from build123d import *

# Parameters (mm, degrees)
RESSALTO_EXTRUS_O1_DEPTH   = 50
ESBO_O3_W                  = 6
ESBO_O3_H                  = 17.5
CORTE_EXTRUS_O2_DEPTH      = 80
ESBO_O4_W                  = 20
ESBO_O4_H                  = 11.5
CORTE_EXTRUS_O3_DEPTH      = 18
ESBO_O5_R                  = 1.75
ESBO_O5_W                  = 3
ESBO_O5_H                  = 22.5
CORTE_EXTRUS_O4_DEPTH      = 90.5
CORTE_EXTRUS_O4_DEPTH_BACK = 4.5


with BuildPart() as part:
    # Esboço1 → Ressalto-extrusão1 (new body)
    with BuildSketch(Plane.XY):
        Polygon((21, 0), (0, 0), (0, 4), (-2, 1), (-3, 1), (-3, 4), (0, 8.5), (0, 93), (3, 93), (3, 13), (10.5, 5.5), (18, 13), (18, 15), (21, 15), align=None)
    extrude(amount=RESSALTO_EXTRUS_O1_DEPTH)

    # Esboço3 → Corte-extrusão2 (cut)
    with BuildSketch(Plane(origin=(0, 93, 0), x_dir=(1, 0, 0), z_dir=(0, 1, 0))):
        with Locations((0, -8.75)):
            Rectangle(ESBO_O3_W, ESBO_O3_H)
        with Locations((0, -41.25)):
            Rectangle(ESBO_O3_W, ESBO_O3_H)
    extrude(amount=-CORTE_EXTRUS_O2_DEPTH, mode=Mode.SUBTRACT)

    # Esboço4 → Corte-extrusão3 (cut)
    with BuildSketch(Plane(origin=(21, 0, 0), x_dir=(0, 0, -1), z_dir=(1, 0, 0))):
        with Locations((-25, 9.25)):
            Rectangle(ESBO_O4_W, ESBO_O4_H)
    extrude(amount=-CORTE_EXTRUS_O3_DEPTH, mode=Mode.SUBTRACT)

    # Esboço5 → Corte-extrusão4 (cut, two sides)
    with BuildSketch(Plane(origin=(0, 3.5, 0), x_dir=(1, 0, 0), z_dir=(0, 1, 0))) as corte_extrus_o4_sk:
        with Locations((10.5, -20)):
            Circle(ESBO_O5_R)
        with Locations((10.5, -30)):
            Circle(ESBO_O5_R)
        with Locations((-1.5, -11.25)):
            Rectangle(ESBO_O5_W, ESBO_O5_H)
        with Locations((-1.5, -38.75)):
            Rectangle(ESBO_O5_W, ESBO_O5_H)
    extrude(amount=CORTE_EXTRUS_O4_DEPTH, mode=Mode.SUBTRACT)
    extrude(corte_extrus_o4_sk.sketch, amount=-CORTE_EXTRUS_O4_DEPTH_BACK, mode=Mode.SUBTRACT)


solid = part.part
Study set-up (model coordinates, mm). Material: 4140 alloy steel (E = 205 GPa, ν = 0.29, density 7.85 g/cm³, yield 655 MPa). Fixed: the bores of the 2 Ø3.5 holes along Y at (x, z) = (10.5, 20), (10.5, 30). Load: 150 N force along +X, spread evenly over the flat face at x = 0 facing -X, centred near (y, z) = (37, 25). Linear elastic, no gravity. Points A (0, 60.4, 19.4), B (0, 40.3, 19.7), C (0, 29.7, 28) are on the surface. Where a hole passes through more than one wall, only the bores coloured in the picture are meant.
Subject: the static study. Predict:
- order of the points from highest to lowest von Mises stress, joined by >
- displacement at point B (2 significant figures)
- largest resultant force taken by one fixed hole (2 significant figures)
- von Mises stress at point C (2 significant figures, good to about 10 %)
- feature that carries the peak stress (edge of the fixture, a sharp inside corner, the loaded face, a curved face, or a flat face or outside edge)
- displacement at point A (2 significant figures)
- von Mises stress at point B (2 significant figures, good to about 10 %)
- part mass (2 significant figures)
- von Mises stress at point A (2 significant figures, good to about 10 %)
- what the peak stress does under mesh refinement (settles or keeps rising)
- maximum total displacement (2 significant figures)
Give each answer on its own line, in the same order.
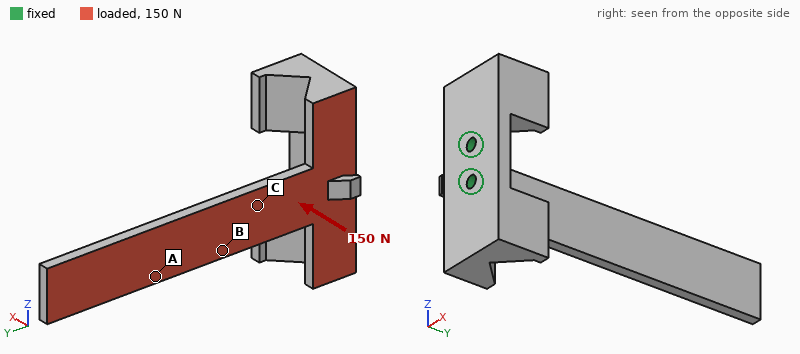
C > B > A
0.29 mm
77 N
110 MPa
a sharp inside corner
0.62 mm
76 MPa
97 g
29 MPa
keeps rising
1.2 mm
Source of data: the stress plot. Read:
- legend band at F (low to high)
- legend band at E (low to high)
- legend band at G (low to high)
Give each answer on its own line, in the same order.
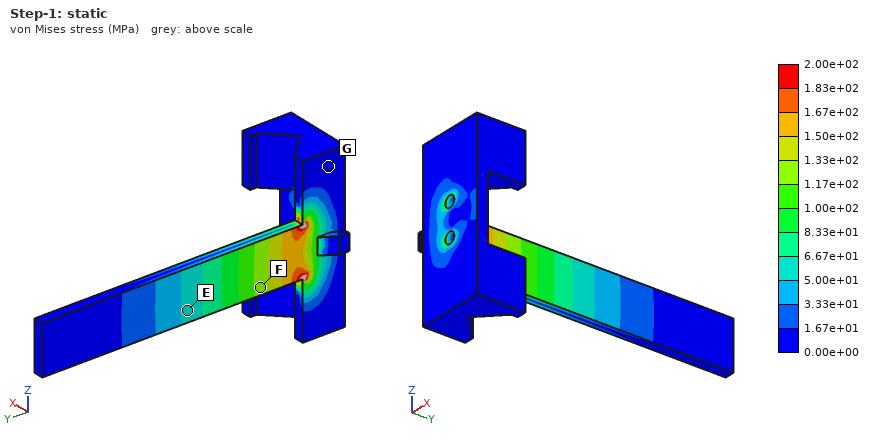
1.17e+02 to 1.33e+02 MPa
5.00e+01 to 6.67e+01 MPa
0.00e+00 to 1.67e+01 MPa
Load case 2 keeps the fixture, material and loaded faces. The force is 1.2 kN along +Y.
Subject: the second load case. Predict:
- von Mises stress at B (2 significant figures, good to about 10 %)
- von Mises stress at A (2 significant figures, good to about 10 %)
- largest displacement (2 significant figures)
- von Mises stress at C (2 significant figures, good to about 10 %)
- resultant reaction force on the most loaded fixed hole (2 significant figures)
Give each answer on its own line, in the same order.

46 MPa
29 MPa
0.56 mm
56 MPa
610 N
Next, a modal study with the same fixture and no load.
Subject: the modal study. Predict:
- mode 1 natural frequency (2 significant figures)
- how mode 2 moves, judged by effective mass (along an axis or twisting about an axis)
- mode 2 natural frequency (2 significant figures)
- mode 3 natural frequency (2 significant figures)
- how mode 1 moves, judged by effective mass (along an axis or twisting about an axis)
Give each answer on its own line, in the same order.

330 Hz
along Z
1300 Hz
2000 Hz
along X
